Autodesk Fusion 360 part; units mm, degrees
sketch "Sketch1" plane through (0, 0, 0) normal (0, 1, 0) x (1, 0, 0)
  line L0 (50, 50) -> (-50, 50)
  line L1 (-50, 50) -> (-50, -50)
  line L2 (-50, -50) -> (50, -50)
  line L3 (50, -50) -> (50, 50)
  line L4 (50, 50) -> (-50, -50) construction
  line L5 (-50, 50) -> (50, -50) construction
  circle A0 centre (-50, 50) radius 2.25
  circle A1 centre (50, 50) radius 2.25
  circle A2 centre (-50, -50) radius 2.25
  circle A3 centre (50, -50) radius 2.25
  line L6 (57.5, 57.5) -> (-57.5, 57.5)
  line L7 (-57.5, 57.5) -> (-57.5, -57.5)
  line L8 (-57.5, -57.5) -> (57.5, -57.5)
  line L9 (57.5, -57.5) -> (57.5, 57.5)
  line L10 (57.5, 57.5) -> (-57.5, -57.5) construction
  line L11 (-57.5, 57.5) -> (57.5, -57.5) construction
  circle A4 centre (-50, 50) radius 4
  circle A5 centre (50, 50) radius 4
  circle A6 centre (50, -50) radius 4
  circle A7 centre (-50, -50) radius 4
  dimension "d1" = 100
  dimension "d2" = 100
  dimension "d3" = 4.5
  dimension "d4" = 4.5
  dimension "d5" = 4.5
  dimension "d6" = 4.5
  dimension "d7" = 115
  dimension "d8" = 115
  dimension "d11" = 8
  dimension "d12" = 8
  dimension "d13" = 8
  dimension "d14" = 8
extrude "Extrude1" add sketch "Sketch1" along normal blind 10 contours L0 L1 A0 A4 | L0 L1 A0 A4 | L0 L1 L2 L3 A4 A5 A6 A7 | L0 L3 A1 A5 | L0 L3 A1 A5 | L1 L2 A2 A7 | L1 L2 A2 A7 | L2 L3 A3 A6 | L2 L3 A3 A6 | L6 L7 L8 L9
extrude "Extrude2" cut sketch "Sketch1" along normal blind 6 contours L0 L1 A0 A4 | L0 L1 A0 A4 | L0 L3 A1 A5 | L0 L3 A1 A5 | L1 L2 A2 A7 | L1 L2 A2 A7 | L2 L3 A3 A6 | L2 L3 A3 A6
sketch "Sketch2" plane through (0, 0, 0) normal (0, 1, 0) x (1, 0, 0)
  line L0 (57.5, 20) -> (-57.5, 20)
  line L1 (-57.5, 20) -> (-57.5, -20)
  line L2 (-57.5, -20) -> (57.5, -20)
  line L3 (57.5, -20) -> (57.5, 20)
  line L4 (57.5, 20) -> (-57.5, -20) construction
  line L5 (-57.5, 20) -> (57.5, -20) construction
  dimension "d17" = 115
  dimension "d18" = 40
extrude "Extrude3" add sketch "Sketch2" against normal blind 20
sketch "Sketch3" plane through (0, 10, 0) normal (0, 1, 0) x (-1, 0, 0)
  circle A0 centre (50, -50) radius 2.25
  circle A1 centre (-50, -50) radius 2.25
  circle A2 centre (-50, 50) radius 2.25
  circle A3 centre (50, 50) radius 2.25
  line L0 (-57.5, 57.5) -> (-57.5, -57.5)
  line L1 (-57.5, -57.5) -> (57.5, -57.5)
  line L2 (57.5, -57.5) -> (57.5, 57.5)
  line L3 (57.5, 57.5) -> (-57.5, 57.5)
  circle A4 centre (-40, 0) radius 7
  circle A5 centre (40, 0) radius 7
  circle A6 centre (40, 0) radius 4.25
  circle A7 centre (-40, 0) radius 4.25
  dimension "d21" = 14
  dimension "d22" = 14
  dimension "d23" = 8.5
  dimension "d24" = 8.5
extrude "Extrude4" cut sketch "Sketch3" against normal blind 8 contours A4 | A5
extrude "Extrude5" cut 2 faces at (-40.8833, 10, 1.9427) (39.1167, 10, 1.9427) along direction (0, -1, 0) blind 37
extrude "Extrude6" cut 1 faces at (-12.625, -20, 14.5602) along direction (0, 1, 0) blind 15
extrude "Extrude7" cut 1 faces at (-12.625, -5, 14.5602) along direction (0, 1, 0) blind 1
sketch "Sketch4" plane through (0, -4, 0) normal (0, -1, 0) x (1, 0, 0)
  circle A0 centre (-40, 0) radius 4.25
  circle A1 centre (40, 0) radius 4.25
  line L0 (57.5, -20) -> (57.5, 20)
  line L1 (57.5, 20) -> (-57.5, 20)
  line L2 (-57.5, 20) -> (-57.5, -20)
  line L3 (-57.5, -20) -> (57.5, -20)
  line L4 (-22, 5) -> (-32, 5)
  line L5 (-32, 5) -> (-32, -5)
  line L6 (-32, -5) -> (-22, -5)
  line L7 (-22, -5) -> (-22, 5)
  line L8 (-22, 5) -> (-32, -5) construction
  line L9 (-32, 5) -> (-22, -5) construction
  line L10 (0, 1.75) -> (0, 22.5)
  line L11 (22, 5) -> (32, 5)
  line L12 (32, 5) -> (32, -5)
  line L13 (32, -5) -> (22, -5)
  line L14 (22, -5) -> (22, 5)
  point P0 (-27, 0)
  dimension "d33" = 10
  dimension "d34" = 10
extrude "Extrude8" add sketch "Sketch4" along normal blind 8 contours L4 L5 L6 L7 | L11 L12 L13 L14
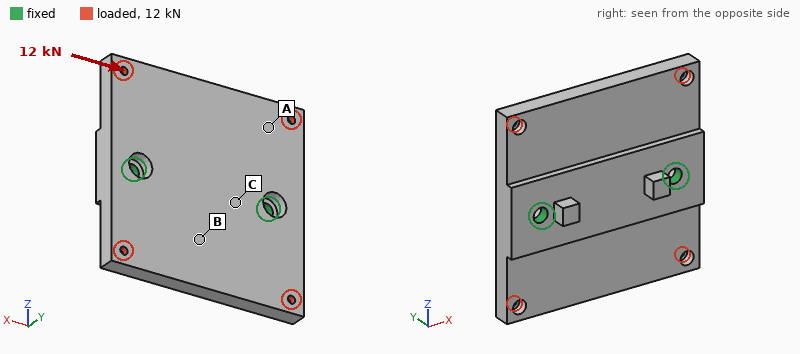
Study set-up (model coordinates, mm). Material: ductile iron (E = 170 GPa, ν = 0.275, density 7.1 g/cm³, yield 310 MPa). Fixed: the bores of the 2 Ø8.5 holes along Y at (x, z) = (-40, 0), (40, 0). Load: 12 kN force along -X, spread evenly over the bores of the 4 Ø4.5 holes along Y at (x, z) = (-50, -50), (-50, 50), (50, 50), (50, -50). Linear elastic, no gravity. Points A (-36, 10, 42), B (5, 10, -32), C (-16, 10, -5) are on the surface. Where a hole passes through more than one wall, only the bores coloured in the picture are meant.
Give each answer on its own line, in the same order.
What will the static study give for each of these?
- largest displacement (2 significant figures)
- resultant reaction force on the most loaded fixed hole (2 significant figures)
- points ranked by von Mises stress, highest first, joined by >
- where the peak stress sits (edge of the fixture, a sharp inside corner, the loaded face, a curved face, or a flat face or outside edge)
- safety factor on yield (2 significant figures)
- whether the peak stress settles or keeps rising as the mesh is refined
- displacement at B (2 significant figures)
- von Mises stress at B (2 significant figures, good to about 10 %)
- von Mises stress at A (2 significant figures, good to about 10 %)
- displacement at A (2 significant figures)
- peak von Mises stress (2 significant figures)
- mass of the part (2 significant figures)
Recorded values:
17 µm
6.1 kN
A > B > C
the loaded face
2.7
settles
4.5 µm
12 MPa
24 MPa
7.5 µm
110 MPa
1.0 kg
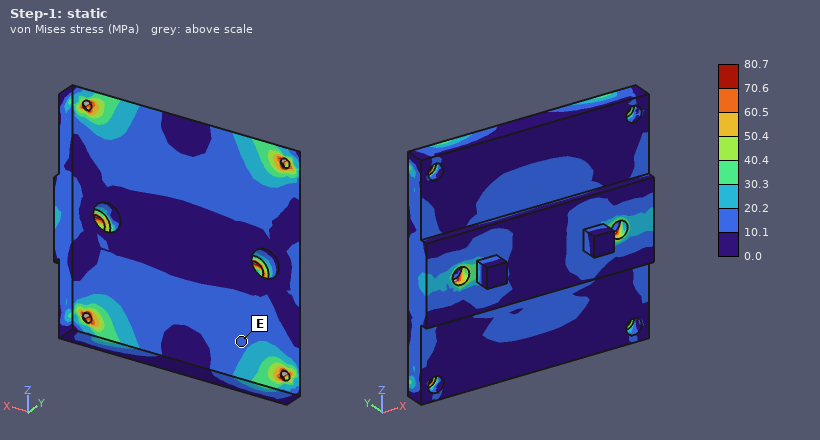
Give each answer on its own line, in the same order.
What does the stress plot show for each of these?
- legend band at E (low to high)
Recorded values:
10.1 to 20.2 MPa
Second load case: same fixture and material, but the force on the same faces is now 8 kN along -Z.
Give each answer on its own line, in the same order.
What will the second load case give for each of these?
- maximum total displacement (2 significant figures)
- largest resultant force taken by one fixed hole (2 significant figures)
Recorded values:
54 µm
4.0 kN
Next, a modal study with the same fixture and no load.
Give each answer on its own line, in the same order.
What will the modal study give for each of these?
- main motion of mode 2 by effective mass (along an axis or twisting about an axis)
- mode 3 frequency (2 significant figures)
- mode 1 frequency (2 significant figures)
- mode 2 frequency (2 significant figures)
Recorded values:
along Y
3300 Hz
1500 Hz
3000 Hz
